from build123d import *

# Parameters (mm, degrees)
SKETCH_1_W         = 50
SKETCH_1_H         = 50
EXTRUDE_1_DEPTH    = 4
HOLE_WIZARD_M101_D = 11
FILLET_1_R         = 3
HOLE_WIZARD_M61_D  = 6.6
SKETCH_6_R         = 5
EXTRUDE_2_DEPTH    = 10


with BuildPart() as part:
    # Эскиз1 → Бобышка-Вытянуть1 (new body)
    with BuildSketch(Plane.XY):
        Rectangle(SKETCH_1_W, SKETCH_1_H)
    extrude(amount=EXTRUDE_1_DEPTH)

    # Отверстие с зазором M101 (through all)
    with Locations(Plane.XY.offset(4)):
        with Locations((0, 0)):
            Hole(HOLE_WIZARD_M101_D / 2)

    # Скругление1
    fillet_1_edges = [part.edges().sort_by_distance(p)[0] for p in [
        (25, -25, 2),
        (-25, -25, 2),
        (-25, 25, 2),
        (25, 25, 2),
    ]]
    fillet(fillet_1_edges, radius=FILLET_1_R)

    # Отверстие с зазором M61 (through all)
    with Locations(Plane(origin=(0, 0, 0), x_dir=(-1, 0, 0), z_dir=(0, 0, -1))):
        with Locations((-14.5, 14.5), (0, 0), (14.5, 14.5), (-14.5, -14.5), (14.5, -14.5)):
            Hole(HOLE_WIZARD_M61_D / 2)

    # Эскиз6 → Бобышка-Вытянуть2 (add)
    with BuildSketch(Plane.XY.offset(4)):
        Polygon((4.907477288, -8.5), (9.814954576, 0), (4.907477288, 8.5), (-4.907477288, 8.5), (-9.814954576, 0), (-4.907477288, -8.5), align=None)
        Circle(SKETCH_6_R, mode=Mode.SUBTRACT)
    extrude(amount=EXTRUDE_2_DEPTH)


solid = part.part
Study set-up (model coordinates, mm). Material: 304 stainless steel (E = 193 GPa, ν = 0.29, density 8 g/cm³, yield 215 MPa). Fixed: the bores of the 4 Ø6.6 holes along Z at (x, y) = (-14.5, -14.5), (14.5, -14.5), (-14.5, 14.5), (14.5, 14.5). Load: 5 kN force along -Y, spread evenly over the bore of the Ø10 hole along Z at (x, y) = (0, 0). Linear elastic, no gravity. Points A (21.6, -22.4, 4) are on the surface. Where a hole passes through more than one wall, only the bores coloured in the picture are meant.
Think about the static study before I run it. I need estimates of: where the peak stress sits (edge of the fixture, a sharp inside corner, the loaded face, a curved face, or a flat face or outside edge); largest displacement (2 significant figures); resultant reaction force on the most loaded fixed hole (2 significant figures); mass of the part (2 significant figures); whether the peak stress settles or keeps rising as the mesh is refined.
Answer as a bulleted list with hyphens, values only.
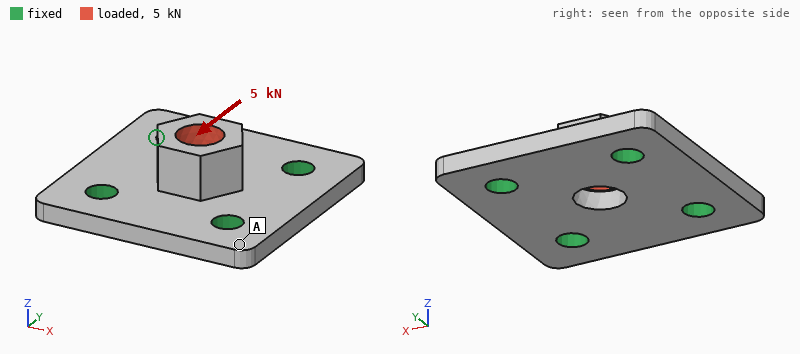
- edge of the fixture
- 18 µm
- 1.5 kN
- 86 g
- keeps rising
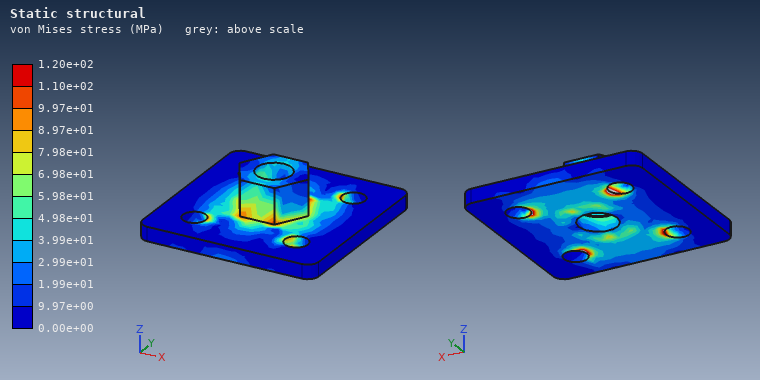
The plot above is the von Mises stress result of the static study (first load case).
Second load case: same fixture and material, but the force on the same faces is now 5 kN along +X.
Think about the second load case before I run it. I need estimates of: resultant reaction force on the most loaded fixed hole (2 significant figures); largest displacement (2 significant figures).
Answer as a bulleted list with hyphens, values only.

- 1.5 kN
- 18 µm
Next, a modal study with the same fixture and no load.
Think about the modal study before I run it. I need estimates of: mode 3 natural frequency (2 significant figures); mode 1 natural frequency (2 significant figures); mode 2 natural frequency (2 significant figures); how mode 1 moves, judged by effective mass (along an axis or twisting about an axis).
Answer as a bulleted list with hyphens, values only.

- 22 kHz
- 19 kHz
- 22 kHz
- along Z
